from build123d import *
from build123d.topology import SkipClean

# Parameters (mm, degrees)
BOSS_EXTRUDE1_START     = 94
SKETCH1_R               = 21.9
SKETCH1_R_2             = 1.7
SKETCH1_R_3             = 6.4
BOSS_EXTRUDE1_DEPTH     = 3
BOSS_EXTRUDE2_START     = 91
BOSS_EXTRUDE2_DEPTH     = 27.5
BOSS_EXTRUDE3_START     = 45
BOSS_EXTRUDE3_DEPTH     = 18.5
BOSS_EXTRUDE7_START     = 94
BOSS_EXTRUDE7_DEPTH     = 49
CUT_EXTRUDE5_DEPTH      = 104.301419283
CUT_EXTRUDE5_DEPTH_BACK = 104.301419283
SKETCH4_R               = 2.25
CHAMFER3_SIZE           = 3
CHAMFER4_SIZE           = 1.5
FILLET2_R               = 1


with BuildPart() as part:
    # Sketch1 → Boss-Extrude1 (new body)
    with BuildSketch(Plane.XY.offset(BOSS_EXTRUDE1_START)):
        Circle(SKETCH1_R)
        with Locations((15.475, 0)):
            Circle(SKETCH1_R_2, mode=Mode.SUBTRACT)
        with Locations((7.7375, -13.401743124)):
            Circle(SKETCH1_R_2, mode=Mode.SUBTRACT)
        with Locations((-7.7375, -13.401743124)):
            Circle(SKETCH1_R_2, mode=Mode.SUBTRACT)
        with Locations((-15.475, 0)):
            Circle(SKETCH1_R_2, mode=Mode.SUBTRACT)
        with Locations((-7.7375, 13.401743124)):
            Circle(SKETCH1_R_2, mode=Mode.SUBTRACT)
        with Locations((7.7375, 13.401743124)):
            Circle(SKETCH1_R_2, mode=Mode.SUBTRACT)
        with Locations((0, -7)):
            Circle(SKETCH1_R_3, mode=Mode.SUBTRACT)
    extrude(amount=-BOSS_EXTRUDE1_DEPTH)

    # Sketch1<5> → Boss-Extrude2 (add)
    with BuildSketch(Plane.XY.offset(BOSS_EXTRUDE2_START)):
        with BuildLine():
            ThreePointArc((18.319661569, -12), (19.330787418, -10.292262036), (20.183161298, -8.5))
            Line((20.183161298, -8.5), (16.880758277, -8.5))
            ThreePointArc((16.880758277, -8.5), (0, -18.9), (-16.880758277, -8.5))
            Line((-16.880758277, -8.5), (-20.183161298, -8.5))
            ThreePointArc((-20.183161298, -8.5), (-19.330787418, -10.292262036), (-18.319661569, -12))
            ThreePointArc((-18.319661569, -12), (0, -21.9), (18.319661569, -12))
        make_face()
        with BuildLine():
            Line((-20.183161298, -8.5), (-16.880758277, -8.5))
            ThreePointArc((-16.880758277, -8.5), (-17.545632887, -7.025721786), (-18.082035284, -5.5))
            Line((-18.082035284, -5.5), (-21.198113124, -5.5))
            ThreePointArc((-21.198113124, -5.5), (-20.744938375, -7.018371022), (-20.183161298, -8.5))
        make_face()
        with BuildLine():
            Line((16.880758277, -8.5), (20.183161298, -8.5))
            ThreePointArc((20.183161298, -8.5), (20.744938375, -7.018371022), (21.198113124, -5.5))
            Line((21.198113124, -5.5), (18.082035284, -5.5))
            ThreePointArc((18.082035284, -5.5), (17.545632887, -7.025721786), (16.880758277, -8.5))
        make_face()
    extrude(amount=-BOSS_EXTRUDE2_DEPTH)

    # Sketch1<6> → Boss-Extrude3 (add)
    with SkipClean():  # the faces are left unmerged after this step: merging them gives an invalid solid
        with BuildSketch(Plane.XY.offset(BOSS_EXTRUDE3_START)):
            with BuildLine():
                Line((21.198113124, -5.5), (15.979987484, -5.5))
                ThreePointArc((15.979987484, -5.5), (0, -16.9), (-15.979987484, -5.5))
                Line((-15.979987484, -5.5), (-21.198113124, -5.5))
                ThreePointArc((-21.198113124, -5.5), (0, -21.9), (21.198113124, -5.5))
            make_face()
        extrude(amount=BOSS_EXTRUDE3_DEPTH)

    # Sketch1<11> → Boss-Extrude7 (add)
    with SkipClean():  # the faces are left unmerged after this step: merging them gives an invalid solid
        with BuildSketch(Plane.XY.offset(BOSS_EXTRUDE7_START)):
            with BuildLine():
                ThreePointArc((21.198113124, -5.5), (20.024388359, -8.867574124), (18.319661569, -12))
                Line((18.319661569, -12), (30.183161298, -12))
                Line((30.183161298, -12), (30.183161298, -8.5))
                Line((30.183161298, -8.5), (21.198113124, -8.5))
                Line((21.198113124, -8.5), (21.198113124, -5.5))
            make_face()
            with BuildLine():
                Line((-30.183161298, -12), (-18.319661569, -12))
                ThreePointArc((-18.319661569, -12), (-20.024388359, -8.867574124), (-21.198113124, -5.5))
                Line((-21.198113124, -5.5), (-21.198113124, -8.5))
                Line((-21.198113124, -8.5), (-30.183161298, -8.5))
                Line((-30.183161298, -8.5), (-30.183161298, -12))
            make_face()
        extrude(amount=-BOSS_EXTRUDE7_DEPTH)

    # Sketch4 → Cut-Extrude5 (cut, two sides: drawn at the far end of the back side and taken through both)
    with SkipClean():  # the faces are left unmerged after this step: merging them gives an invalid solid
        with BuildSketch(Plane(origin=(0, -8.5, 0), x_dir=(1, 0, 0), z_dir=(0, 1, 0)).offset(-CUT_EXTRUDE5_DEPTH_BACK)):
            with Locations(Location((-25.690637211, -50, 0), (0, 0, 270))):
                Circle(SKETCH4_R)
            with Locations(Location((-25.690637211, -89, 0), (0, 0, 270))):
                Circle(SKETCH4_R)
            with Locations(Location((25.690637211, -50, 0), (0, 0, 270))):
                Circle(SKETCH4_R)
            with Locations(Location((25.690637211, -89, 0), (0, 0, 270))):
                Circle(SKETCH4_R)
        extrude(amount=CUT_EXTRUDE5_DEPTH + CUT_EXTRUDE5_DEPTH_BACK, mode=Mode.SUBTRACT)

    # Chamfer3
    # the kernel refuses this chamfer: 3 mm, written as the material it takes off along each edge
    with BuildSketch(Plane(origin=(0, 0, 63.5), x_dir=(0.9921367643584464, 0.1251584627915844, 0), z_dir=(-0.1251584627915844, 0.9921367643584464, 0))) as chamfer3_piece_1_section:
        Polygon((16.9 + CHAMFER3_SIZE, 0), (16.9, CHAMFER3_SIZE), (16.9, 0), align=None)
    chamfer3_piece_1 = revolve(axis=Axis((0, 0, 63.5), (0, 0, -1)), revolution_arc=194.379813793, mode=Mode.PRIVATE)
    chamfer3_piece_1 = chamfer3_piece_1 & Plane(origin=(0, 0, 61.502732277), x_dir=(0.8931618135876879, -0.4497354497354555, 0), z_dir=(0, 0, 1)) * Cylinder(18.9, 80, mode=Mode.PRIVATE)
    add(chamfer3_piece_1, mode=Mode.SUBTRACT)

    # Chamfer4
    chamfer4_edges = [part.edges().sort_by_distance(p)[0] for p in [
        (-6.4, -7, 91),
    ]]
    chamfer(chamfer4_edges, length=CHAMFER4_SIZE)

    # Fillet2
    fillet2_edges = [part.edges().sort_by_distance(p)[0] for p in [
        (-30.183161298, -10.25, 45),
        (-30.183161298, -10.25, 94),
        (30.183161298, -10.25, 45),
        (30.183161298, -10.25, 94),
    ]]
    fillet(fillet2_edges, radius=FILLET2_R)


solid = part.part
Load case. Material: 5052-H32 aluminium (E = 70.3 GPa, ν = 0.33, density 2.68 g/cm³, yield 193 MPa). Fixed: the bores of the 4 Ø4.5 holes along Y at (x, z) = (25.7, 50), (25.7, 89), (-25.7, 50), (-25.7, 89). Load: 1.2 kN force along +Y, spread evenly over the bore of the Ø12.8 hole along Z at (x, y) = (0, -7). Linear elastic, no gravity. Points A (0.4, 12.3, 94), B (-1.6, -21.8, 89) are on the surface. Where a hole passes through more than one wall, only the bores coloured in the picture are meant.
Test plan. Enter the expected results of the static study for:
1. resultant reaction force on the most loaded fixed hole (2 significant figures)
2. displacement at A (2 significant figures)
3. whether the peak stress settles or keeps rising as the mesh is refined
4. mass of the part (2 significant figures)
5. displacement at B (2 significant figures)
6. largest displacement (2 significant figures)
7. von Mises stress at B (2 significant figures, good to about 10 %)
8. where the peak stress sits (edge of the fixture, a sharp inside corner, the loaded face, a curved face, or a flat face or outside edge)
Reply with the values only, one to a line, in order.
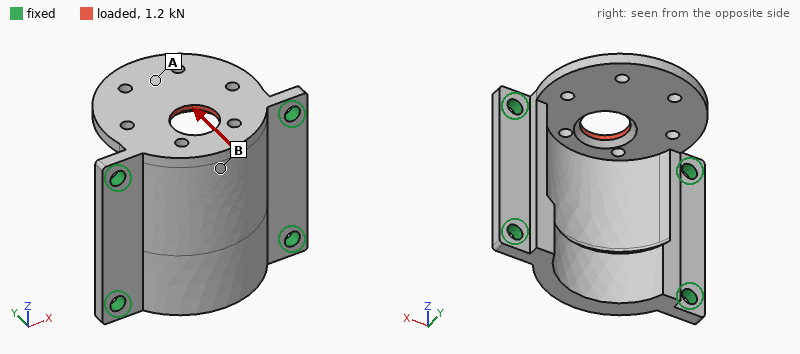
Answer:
650 N
51 µm
keeps rising
44 g
15 µm
69 µm
14 MPa
edge of the fixture
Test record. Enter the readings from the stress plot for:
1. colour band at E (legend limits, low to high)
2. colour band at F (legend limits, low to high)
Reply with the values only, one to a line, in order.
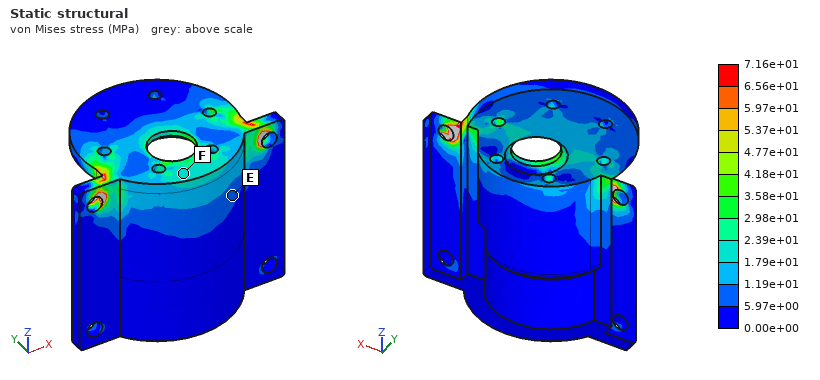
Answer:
5.97e+00 to 1.19e+01 MPa
1.79e+01 to 2.39e+01 MPa
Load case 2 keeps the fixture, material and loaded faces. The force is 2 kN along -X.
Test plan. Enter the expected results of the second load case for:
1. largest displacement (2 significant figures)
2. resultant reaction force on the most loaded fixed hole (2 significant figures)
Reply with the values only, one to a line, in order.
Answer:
13 µm
970 N
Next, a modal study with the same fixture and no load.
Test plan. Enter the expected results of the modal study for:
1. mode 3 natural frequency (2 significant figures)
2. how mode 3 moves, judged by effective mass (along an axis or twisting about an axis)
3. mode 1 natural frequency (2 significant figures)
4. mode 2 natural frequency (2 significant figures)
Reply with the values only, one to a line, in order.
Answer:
11 kHz
along Y
2400 Hz
7000 Hz
